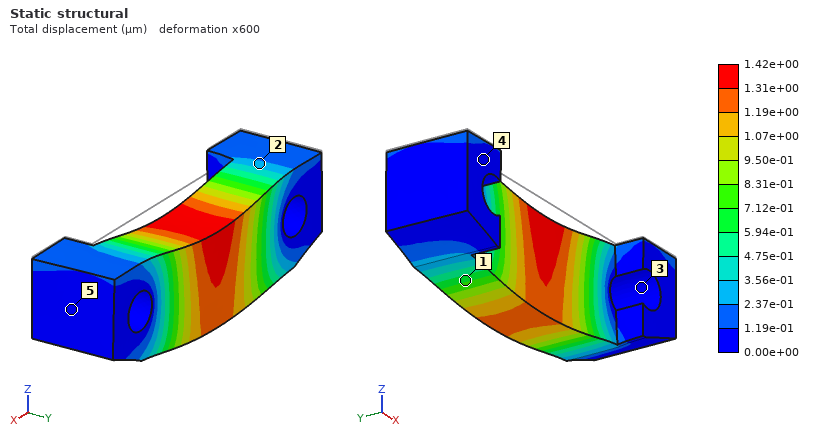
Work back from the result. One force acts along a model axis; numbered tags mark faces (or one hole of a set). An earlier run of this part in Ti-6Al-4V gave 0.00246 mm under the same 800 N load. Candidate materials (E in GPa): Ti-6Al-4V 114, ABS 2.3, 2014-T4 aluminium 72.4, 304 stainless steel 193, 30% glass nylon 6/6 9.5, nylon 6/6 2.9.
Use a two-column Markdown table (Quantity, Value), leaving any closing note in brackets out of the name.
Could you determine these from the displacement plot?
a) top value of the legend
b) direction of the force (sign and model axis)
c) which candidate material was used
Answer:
| Quantity | Value |
|---|---|
| top value of the legend | 1.42e+00 µm |
| direction of the force | -Z |
| which candidate material was used | 304 stainless steel |
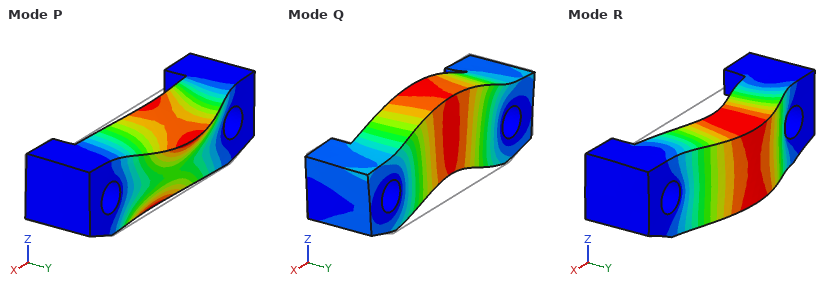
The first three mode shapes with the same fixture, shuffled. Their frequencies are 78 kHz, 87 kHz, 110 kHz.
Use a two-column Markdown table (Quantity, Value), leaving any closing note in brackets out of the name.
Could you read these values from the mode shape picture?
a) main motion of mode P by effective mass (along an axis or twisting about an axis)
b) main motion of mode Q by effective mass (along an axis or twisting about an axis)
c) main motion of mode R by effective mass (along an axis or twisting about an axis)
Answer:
| Quantity | Value |
|---|---|
| main motion of mode P by effective mass | twisting about X |
| main motion of mode Q by effective mass | along Z |
| main motion of mode R by effective mass | along Y |
